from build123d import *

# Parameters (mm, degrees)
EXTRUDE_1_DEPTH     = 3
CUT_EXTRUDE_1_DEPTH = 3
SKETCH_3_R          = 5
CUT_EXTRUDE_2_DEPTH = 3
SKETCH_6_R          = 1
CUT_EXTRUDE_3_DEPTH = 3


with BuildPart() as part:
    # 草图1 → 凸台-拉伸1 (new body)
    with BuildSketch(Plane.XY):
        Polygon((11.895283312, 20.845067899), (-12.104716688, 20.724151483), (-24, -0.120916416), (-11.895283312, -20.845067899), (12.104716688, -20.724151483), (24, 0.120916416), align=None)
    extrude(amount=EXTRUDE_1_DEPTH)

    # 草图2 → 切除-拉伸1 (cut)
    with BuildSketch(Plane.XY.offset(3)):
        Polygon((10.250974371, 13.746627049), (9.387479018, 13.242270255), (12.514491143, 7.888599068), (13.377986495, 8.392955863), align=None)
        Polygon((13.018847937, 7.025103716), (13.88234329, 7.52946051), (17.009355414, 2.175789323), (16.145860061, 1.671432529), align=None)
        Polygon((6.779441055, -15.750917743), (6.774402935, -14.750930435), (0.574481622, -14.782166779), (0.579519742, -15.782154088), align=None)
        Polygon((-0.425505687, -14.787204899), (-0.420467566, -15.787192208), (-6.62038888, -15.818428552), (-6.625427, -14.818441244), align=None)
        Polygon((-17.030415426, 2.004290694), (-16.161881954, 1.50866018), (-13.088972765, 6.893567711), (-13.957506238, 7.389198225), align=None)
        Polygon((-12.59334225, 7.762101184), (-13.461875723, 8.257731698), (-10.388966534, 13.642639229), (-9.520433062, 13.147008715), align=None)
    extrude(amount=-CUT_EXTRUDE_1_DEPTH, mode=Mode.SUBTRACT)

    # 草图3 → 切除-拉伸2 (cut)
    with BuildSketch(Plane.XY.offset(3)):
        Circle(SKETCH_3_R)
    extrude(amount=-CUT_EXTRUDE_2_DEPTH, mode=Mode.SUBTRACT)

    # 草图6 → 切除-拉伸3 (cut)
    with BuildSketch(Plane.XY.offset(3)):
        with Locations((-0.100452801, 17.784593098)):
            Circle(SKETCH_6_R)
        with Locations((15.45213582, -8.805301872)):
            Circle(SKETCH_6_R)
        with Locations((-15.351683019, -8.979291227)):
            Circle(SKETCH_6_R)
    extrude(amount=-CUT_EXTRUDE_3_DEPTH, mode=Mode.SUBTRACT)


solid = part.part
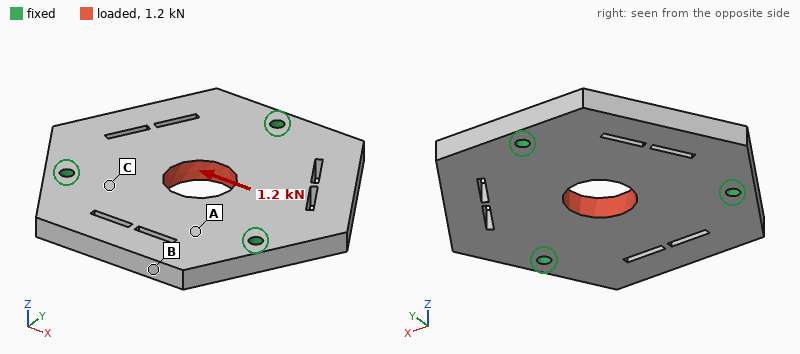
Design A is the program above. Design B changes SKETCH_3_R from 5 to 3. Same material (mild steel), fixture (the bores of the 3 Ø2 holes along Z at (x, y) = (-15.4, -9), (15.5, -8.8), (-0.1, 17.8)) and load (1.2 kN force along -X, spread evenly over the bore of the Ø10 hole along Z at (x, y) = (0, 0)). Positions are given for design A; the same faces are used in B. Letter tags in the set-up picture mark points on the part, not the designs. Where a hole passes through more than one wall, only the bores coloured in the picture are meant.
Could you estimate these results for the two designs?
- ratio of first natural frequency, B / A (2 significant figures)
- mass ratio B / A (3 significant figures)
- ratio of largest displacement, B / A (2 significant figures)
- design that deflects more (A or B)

1.0
1.04
1.1
B
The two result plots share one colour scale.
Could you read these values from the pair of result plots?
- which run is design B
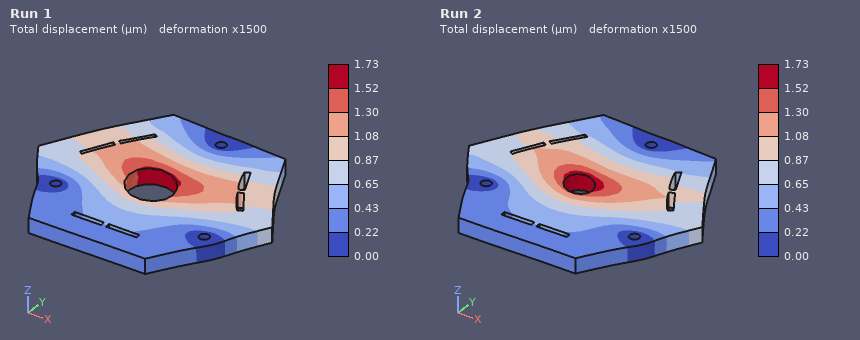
Run 2
